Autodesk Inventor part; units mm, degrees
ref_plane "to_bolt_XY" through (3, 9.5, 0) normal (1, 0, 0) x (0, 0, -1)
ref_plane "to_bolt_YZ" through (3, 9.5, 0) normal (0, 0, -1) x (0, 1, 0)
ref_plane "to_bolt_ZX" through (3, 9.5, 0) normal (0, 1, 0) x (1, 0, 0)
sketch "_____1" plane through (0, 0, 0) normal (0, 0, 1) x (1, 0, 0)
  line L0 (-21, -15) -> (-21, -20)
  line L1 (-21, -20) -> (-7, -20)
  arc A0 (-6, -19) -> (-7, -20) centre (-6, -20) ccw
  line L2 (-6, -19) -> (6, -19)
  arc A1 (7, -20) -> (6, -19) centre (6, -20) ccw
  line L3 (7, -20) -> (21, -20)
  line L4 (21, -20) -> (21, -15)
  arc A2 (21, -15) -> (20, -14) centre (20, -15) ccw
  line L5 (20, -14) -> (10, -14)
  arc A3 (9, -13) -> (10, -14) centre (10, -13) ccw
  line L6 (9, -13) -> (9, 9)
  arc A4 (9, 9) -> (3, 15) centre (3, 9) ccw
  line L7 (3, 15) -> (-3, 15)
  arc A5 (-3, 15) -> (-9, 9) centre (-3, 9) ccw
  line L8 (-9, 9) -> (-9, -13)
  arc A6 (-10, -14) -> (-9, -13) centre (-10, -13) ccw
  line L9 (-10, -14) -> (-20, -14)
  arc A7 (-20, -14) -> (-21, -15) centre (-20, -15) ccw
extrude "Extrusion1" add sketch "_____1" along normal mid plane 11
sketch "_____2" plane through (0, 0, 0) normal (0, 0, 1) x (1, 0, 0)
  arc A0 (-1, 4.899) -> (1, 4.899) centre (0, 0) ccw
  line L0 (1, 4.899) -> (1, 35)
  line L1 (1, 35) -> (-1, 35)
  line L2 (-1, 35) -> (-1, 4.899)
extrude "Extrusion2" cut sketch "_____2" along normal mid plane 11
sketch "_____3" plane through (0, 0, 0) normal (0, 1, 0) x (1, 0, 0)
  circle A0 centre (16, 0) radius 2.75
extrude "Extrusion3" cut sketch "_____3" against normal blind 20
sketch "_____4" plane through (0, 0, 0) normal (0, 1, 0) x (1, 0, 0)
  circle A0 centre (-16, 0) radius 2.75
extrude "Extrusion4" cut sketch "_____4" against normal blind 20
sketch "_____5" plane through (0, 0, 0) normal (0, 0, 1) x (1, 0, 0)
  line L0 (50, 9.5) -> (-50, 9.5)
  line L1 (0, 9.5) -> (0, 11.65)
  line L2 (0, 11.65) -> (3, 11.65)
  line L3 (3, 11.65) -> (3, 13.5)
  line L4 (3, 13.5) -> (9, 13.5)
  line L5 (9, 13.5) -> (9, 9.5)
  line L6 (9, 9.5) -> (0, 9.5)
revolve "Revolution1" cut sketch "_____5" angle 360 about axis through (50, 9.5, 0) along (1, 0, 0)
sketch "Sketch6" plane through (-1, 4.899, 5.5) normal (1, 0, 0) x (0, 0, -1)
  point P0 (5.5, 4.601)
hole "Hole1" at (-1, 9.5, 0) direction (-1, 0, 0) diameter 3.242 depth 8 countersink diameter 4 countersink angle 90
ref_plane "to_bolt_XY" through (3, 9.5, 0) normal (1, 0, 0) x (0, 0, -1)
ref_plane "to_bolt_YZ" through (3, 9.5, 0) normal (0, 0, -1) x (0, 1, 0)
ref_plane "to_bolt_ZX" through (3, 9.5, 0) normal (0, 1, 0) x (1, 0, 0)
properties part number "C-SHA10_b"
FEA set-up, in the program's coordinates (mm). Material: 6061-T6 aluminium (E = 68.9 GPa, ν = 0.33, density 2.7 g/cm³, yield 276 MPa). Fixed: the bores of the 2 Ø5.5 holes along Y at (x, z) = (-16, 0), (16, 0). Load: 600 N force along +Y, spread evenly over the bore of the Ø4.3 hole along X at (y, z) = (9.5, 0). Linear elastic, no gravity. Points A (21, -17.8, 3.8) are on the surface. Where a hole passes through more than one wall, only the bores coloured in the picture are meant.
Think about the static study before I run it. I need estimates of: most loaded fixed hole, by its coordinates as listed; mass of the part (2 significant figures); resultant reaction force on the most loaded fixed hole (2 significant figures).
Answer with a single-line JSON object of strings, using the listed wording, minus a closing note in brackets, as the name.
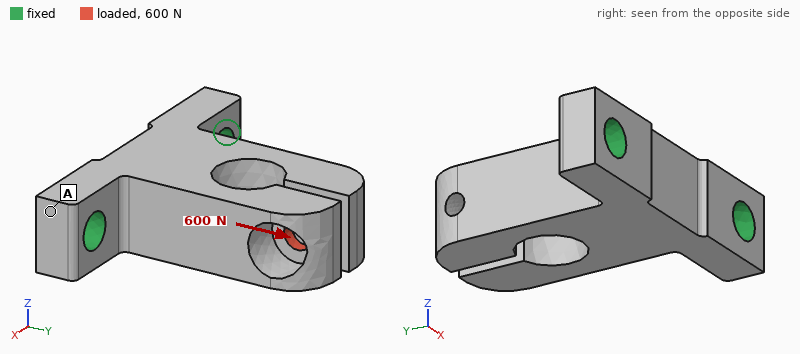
{"most loaded fixed hole, by its coordinates as listed": "(16, 0)", "mass of the part": "17 g", "resultant reaction force on the most loaded fixed hole": "390 N"}
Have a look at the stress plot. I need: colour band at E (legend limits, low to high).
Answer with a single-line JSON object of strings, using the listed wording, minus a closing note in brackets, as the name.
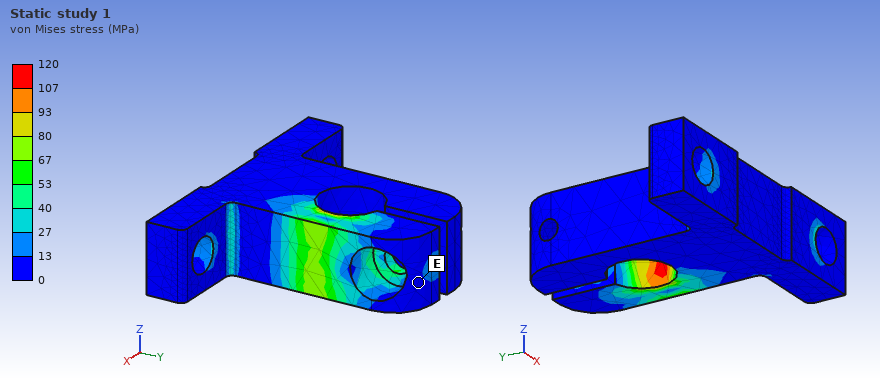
{"colour band at E": "0 to 13 MPa"}
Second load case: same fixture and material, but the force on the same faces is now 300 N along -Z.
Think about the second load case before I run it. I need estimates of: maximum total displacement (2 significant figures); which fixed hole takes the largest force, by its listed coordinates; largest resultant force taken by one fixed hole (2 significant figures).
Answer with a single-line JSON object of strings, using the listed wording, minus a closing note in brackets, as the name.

{"maximum total displacement": "0.12 mm", "which fixed hole takes the largest force, by its listed coordinates": "(16, 0)", "largest resultant force taken by one fixed hole": "170 N"}
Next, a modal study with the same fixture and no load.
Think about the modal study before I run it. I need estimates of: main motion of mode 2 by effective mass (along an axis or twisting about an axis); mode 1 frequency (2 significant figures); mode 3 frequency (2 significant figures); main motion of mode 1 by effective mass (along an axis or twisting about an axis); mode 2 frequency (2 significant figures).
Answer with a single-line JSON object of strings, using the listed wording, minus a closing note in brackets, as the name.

{"main motion of mode 2 by effective mass": "along X", "mode 1 frequency": "4800 Hz", "mode 3 frequency": "7600 Hz", "main motion of mode 1 by effective mass": "along Z", "mode 2 frequency": "6400 Hz"}
